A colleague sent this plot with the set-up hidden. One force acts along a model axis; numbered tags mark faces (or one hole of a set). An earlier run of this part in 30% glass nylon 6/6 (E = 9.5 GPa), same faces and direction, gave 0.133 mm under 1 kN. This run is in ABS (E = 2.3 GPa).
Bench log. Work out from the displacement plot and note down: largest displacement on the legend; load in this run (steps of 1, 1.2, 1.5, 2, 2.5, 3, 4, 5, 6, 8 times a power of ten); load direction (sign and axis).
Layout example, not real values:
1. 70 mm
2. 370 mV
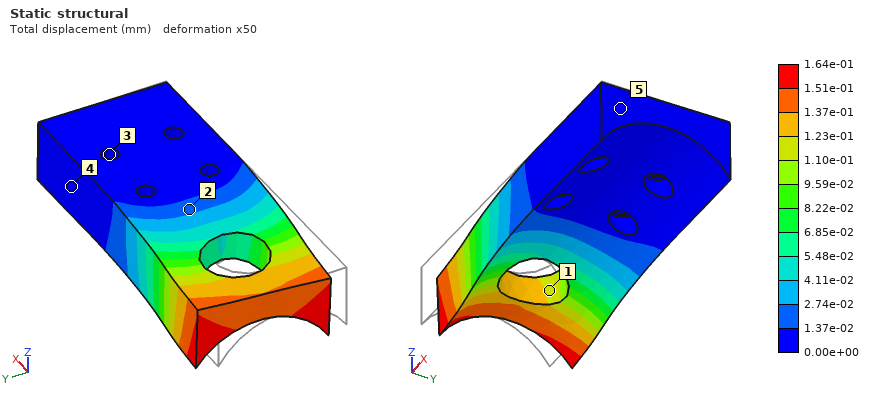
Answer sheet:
1. 1.64e-01 mm
2. 300 N
3. +Y
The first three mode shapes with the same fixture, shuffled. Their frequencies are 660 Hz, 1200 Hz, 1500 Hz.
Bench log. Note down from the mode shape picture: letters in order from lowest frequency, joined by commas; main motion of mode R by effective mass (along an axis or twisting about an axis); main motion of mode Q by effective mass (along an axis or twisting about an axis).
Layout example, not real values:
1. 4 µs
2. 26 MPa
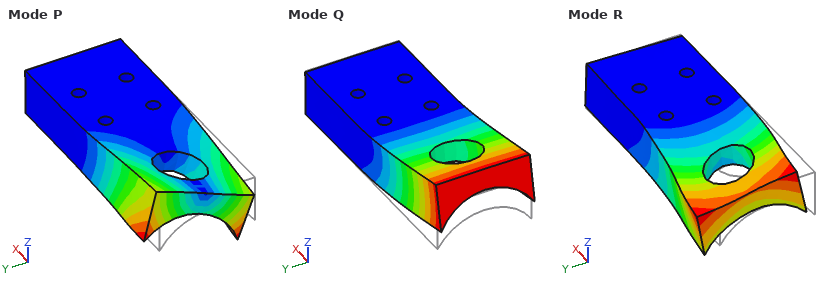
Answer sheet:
1. Q, P, R
2. along Y
3. along Z
